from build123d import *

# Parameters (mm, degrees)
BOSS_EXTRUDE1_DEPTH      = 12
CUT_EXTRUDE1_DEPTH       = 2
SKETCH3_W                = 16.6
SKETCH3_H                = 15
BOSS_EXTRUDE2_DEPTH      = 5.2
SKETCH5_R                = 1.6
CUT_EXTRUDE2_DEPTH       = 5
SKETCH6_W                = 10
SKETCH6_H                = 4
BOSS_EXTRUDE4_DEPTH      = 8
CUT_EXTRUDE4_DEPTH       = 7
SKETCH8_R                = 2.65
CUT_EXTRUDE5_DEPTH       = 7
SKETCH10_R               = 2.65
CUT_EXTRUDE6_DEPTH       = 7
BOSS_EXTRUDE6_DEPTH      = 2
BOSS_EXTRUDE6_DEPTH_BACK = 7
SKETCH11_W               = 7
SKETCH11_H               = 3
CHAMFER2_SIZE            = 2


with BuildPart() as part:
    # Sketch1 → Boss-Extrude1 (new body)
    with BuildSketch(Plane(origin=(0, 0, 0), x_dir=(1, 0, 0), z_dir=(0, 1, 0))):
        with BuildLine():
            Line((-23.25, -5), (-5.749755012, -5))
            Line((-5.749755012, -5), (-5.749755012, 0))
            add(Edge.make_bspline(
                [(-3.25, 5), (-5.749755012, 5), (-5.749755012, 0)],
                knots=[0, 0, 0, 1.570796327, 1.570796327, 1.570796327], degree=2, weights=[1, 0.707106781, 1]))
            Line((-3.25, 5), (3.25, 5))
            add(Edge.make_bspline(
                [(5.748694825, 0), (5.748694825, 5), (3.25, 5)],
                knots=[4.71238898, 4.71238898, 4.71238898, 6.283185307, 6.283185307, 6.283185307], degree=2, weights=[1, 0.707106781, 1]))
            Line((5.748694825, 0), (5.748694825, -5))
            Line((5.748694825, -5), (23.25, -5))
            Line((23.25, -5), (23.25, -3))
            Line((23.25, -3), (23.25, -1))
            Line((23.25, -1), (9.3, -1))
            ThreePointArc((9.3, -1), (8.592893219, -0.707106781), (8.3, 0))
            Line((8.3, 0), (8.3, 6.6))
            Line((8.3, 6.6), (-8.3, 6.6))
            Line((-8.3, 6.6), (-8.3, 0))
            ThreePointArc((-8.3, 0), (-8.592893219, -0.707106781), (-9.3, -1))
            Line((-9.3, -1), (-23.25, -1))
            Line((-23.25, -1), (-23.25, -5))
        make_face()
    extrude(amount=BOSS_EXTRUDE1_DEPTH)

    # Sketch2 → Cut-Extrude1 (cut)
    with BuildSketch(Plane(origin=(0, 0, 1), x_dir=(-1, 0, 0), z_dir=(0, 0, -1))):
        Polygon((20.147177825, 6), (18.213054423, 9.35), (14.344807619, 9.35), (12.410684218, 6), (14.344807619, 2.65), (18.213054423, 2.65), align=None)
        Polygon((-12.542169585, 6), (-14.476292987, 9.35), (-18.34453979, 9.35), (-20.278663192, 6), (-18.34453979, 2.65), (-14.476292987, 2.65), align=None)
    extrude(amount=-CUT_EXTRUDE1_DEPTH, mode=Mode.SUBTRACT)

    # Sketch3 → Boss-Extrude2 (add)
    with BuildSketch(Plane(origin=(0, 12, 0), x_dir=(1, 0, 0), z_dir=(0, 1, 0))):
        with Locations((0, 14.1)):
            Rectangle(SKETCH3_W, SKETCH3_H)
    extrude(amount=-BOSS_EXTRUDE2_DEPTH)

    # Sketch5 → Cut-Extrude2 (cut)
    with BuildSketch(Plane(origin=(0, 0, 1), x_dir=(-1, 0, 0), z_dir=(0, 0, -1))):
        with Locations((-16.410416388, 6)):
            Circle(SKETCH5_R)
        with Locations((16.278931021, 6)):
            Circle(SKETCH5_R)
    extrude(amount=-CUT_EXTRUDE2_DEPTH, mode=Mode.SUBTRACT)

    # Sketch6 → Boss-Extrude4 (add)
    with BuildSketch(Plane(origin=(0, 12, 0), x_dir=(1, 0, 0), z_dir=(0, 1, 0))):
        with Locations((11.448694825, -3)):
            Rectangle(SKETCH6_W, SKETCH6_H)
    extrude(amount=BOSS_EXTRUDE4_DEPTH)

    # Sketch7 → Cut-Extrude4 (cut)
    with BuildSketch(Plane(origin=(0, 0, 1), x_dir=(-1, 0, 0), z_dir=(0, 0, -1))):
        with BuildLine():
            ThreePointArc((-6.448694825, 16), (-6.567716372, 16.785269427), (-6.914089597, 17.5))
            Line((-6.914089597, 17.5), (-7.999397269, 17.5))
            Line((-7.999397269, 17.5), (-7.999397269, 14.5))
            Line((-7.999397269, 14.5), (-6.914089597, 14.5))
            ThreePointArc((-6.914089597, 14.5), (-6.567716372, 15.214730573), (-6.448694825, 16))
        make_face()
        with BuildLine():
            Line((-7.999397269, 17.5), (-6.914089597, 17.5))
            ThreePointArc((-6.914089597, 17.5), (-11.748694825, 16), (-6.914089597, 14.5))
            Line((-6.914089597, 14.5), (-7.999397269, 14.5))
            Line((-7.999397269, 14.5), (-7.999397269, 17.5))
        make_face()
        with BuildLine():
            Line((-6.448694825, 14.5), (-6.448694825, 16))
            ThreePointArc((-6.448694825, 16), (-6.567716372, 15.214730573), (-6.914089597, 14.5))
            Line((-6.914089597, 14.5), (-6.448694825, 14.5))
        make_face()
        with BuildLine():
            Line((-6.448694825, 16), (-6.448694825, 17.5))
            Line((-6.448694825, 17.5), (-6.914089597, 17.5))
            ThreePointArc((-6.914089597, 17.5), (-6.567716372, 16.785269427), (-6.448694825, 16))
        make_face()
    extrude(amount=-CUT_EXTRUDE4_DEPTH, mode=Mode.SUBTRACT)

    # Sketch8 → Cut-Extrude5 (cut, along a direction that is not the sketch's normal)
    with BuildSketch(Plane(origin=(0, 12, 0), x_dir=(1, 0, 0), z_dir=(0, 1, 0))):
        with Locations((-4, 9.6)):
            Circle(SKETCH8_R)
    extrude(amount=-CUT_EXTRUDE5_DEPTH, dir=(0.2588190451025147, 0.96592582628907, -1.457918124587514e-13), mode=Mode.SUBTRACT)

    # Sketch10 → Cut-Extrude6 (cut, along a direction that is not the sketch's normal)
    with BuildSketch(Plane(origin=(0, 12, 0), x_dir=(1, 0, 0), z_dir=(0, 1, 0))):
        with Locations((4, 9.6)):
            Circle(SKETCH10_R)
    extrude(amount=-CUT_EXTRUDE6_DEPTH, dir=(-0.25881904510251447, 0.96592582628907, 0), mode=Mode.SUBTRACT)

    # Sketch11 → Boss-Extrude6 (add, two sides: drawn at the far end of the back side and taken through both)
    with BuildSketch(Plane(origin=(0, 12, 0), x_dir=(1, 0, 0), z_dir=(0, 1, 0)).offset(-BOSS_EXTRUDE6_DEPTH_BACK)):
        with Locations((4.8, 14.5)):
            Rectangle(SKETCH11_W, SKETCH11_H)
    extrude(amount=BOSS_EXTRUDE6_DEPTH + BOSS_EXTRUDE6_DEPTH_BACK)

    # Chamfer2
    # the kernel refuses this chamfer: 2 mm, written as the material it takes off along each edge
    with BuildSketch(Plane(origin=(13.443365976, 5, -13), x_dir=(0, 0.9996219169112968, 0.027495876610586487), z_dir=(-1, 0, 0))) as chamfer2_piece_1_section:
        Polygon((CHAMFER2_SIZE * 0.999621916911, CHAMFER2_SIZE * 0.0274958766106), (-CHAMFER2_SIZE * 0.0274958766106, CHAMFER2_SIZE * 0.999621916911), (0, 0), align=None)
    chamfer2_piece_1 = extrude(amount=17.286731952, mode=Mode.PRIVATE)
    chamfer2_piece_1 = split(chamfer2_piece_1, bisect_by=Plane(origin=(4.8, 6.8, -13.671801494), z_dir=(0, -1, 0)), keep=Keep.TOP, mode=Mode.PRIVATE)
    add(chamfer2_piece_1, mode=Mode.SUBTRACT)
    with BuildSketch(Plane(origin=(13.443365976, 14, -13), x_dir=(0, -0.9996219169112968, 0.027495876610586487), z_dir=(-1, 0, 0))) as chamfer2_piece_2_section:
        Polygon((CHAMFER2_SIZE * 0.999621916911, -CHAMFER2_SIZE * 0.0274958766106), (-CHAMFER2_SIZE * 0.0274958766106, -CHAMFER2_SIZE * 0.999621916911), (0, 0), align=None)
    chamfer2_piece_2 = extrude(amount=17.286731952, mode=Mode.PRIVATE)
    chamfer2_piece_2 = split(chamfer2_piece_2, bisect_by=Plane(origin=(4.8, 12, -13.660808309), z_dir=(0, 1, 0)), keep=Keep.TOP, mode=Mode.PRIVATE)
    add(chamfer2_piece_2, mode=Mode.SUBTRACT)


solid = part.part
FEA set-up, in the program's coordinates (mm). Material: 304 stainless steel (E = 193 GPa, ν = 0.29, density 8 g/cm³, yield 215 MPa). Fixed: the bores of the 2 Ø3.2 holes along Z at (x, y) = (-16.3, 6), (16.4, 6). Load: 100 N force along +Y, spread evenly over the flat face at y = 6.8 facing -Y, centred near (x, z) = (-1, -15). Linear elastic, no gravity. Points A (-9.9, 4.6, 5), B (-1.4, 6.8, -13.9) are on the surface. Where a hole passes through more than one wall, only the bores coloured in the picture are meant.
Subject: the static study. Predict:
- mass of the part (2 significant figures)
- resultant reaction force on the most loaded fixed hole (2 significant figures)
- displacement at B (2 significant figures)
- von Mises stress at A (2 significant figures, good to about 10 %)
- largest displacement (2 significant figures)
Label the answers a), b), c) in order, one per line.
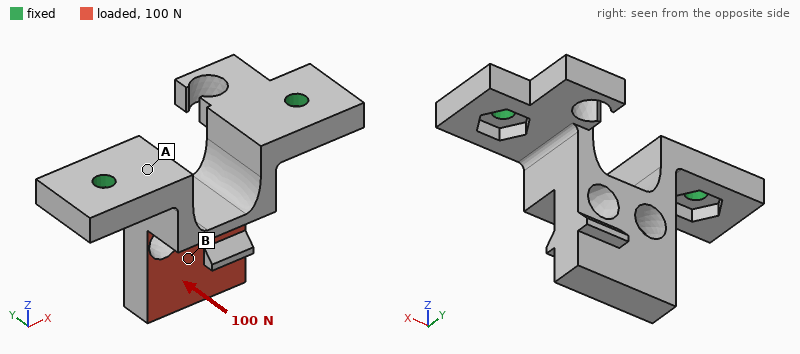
a) 29 g
b) 51 N
c) 20 µm
d) 24 MPa
e) 32 µm
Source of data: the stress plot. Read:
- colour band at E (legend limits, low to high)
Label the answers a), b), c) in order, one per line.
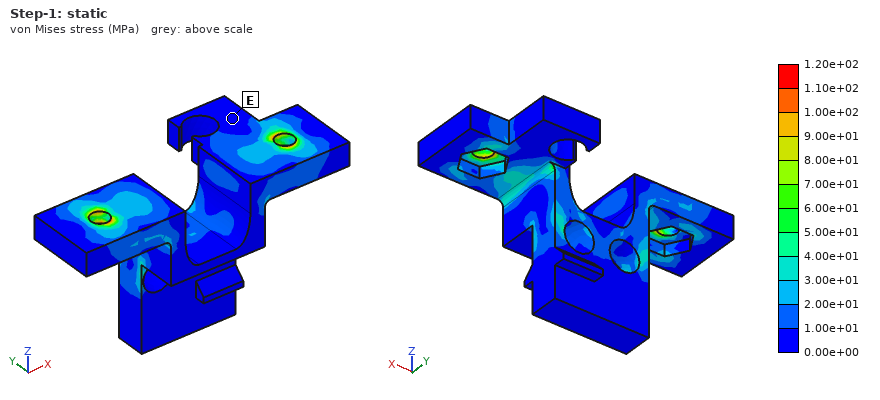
a) 0.00e+00 to 1.00e+01 MPa
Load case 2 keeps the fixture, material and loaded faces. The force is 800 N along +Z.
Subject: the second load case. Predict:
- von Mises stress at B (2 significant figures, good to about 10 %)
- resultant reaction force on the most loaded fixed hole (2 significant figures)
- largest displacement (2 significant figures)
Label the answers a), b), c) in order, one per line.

a) 40 MPa
b) 530 N
c) 16 µm
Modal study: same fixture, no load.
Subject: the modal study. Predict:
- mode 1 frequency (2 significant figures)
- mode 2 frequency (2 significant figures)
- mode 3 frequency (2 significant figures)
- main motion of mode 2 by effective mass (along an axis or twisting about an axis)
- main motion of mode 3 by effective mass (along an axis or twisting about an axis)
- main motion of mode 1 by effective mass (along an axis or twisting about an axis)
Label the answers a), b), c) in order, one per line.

a) 3200 Hz
b) 7500 Hz
c) 11 kHz
d) along X
e) along Z
f) along Y
